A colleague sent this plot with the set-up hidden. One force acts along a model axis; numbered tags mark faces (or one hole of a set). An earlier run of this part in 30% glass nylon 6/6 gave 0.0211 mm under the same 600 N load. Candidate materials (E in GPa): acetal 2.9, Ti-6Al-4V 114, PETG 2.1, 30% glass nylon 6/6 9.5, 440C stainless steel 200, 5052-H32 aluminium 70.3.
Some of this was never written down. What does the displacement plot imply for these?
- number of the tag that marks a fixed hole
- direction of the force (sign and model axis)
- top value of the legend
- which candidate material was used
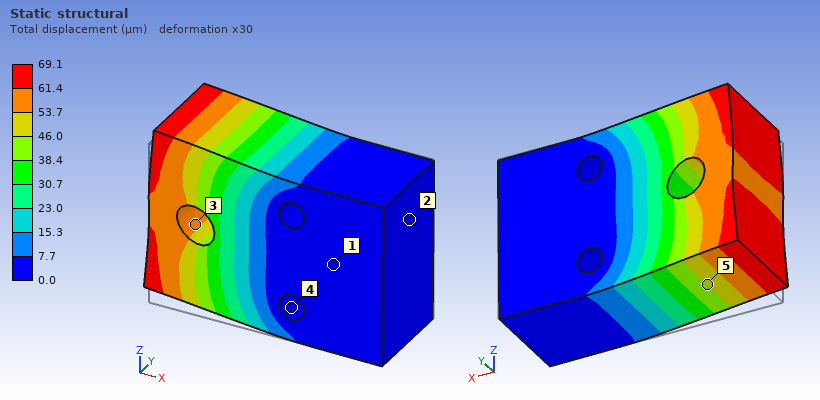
4
+Z
69.1 µm
acetal
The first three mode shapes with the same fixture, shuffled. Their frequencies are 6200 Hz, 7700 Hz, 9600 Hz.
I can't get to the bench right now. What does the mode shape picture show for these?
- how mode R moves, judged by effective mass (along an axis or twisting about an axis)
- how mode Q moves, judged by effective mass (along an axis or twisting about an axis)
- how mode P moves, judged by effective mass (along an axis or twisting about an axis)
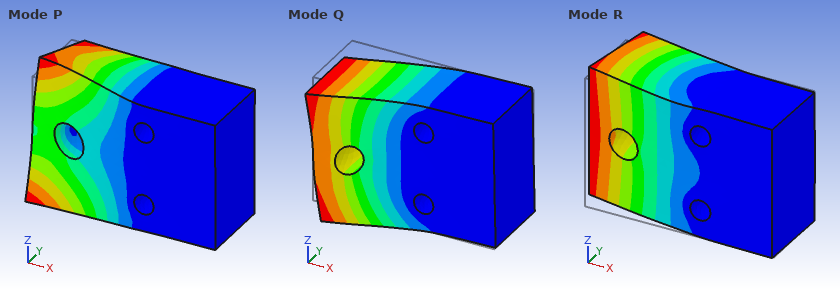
along Y
along Z
twisting about X
